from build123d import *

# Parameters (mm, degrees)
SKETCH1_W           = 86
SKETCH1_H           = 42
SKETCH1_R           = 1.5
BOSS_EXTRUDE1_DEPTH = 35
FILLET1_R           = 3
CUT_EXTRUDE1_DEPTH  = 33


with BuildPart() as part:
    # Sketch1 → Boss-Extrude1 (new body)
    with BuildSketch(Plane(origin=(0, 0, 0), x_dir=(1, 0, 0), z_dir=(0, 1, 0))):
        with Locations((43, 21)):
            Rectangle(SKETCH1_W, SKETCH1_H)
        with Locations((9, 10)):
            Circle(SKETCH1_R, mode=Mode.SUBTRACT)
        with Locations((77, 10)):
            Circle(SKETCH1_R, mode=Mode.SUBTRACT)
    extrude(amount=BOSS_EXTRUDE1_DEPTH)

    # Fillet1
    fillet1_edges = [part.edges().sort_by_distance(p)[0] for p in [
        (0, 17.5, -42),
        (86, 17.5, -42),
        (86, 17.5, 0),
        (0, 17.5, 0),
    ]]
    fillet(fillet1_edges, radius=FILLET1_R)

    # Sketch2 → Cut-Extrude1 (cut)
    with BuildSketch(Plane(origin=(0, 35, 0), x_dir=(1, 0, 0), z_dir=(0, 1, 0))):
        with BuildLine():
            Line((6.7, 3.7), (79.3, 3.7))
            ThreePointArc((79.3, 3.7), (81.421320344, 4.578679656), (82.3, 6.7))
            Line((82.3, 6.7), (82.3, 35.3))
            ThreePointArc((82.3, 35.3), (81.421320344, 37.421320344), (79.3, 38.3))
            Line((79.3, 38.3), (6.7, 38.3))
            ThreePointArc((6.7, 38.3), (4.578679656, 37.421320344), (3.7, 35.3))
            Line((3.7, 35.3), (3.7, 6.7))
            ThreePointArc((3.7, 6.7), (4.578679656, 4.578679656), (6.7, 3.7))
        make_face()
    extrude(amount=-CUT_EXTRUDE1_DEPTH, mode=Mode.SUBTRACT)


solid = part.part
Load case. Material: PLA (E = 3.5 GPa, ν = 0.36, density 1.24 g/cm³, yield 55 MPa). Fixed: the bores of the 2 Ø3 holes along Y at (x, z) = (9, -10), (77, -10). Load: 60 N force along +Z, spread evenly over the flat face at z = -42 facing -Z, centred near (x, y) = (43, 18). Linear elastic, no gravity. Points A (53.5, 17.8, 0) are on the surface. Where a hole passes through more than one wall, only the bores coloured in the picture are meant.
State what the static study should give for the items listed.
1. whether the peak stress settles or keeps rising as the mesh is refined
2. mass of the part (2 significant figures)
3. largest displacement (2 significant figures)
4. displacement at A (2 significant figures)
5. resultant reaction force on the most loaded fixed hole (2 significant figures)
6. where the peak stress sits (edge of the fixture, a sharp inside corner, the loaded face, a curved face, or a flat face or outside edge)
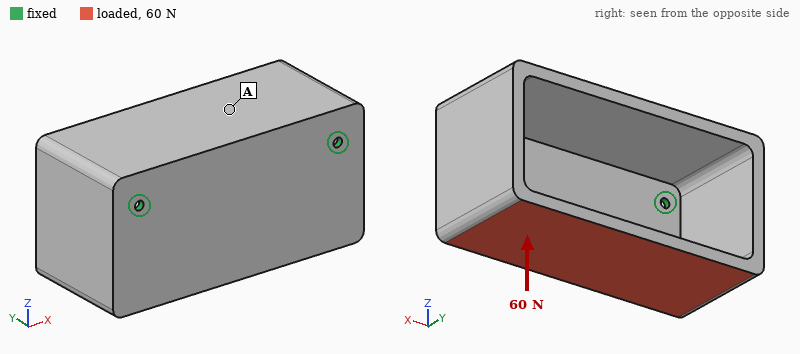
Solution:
keeps rising
45 g
1.1 mm
0.39 mm
30 N
edge of the fixture
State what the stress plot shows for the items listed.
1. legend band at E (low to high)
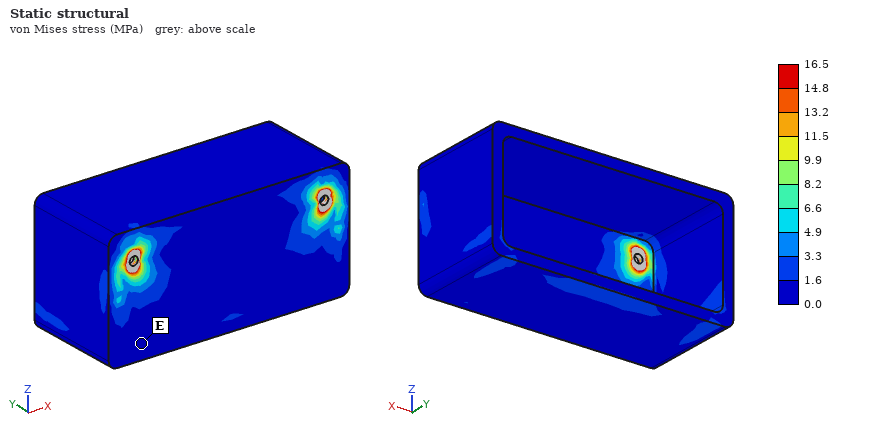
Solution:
0.0 to 1.6 MPa
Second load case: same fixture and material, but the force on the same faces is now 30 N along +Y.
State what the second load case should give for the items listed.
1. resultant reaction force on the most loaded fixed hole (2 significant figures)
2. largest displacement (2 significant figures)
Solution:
15 N
0.98 mm
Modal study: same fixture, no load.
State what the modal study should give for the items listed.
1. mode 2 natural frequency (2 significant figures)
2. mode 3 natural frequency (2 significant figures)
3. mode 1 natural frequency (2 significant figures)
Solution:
580 Hz
1000 Hz
190 Hz
